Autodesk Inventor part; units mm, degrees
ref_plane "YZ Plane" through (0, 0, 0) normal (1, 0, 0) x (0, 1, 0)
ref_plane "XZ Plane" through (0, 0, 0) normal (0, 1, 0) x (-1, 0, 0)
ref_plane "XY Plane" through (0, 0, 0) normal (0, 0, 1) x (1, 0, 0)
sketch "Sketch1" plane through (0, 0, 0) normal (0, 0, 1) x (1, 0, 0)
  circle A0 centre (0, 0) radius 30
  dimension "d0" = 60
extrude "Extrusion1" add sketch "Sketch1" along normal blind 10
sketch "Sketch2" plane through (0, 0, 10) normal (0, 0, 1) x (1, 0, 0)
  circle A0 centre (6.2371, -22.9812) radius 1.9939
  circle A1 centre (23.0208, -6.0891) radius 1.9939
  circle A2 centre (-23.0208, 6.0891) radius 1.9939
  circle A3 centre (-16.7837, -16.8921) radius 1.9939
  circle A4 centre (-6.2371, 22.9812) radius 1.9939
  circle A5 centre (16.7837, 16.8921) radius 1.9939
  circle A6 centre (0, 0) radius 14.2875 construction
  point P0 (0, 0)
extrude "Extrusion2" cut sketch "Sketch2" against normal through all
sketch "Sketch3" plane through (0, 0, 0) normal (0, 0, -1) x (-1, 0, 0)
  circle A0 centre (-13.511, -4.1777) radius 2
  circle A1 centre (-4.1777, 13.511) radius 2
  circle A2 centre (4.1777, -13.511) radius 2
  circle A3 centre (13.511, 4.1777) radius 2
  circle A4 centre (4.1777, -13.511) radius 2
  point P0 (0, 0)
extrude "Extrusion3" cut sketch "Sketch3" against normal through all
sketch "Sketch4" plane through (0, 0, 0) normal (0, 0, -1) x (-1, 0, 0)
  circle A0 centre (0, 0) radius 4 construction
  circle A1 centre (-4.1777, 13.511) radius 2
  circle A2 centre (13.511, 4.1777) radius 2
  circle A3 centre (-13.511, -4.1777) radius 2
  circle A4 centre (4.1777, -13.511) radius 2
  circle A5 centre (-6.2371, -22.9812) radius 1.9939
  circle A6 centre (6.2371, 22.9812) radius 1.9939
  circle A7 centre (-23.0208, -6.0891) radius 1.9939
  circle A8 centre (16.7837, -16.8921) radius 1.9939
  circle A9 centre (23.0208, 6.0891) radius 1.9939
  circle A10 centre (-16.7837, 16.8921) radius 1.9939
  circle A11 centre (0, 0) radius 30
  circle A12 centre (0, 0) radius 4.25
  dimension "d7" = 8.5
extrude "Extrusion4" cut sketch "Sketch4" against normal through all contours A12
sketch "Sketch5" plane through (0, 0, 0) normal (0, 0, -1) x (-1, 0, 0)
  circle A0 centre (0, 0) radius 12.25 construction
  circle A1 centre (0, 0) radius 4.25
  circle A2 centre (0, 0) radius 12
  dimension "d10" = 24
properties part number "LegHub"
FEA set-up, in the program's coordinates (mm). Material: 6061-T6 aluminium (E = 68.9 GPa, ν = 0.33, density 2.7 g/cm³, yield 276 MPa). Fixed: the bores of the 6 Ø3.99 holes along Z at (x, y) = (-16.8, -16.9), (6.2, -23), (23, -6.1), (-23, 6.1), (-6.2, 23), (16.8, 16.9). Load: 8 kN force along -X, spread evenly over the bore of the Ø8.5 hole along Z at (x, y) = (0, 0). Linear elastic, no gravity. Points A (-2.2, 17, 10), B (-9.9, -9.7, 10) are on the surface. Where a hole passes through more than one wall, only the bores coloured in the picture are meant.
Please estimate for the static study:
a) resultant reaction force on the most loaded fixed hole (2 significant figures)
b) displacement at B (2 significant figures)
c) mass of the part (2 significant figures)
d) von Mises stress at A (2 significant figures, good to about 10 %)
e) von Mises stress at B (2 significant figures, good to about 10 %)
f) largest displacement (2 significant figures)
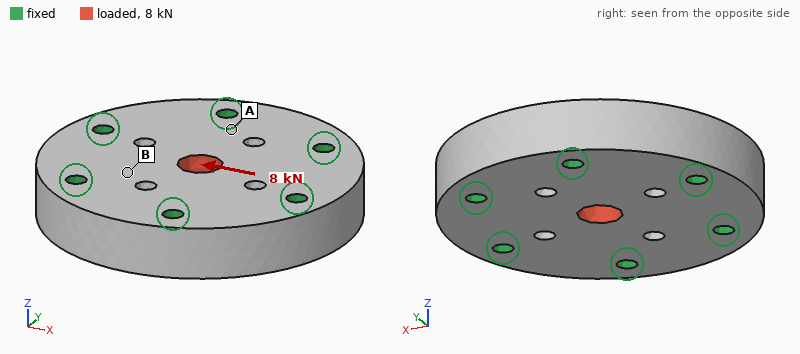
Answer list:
1.9 kN
2.4 µm
71 g
5.7 MPa
15 MPa
6.7 µm
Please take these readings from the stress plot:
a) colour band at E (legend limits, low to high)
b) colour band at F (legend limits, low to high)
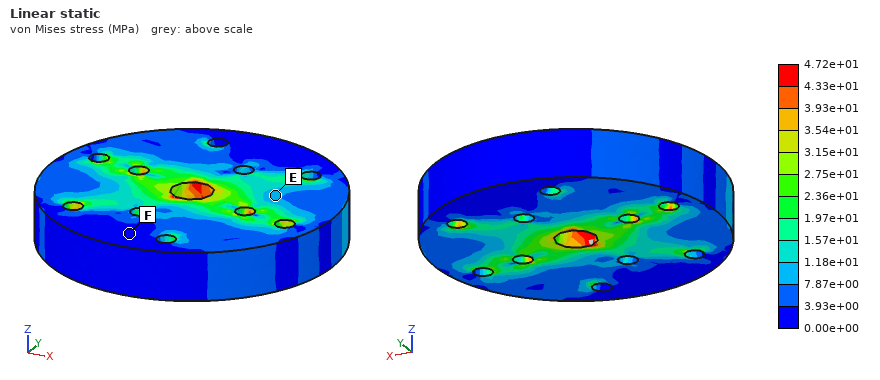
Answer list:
7.87e+00 to 1.18e+01 MPa
0.00e+00 to 3.93e+00 MPa
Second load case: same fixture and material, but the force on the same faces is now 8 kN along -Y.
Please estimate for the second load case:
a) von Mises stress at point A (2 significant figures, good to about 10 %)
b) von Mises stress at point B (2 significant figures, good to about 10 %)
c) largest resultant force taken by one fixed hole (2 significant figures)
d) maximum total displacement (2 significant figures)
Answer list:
19 MPa
14 MPa
2.1 kN
6.3 µm
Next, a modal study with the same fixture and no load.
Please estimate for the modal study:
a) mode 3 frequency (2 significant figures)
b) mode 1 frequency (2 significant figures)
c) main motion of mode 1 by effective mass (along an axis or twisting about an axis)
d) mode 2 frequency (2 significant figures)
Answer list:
44 kHz
27 kHz
along Z
44 kHz
